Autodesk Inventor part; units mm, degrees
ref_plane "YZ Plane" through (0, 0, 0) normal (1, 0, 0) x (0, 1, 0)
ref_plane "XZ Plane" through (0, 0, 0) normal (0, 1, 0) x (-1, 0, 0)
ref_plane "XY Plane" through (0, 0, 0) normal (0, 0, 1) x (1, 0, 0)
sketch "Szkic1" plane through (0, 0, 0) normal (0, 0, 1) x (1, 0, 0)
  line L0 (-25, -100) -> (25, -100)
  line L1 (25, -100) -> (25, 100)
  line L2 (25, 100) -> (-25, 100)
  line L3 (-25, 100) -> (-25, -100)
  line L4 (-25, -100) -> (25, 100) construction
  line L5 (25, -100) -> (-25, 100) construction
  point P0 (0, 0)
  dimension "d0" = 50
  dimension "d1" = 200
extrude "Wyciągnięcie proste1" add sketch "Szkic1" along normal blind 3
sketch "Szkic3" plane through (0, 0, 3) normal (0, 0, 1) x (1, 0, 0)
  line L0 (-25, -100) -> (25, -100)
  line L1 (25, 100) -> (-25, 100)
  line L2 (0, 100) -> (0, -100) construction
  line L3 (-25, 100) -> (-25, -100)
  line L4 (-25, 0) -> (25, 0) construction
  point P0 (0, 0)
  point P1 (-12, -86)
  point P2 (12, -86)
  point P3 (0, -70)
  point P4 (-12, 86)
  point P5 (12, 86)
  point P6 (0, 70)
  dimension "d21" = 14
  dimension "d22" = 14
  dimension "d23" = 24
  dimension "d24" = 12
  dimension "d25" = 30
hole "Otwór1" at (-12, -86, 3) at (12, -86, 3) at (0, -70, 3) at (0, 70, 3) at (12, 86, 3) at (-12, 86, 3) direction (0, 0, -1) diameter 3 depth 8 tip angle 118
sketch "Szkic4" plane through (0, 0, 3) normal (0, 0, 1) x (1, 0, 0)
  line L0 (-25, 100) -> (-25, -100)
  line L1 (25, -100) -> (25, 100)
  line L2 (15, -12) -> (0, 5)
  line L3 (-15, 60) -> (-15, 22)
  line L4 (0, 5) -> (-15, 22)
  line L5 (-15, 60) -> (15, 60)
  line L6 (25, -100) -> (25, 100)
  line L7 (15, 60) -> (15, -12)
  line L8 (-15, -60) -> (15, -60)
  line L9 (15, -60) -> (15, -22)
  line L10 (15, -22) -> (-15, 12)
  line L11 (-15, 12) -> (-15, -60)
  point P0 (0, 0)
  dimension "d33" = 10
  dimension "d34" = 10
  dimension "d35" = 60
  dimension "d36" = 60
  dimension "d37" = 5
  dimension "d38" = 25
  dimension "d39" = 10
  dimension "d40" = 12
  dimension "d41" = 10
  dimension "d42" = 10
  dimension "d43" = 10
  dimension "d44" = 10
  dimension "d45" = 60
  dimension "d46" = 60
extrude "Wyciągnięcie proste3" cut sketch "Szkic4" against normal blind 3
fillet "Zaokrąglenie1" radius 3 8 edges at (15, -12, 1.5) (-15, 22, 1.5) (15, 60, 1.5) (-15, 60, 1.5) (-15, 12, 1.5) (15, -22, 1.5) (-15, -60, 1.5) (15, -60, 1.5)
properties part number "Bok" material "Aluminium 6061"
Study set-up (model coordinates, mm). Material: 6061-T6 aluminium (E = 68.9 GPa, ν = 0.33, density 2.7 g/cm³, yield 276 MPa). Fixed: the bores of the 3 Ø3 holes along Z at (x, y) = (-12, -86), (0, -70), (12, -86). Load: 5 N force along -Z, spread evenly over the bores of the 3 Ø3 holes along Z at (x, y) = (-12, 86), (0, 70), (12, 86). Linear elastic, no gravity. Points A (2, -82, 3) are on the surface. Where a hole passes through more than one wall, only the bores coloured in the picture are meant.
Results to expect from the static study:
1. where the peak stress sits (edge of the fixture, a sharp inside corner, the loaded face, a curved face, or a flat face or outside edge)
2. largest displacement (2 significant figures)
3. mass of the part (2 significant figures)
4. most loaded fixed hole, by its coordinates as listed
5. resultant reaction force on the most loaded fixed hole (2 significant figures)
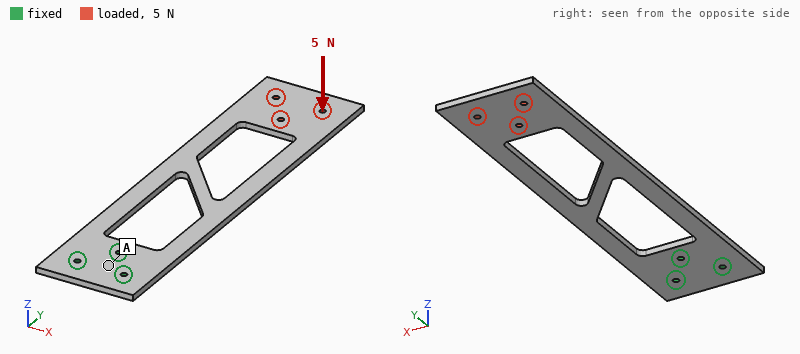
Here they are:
a curved face
2.1 mm
54 g
(0, -70)
36 N
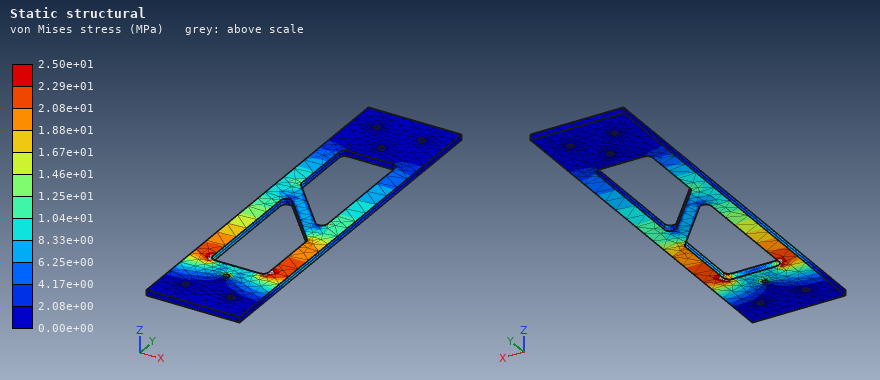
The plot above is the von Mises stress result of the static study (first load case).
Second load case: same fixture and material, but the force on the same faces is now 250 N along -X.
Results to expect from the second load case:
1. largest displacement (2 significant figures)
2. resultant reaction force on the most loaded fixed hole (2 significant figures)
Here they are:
0.62 mm
1.1 kN
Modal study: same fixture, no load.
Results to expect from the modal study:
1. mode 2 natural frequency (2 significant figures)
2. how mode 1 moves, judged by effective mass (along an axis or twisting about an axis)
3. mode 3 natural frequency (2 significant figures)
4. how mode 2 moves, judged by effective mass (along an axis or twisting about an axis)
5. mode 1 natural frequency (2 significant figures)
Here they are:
370 Hz
along Z
450 Hz
twisting about Y
62 Hz
